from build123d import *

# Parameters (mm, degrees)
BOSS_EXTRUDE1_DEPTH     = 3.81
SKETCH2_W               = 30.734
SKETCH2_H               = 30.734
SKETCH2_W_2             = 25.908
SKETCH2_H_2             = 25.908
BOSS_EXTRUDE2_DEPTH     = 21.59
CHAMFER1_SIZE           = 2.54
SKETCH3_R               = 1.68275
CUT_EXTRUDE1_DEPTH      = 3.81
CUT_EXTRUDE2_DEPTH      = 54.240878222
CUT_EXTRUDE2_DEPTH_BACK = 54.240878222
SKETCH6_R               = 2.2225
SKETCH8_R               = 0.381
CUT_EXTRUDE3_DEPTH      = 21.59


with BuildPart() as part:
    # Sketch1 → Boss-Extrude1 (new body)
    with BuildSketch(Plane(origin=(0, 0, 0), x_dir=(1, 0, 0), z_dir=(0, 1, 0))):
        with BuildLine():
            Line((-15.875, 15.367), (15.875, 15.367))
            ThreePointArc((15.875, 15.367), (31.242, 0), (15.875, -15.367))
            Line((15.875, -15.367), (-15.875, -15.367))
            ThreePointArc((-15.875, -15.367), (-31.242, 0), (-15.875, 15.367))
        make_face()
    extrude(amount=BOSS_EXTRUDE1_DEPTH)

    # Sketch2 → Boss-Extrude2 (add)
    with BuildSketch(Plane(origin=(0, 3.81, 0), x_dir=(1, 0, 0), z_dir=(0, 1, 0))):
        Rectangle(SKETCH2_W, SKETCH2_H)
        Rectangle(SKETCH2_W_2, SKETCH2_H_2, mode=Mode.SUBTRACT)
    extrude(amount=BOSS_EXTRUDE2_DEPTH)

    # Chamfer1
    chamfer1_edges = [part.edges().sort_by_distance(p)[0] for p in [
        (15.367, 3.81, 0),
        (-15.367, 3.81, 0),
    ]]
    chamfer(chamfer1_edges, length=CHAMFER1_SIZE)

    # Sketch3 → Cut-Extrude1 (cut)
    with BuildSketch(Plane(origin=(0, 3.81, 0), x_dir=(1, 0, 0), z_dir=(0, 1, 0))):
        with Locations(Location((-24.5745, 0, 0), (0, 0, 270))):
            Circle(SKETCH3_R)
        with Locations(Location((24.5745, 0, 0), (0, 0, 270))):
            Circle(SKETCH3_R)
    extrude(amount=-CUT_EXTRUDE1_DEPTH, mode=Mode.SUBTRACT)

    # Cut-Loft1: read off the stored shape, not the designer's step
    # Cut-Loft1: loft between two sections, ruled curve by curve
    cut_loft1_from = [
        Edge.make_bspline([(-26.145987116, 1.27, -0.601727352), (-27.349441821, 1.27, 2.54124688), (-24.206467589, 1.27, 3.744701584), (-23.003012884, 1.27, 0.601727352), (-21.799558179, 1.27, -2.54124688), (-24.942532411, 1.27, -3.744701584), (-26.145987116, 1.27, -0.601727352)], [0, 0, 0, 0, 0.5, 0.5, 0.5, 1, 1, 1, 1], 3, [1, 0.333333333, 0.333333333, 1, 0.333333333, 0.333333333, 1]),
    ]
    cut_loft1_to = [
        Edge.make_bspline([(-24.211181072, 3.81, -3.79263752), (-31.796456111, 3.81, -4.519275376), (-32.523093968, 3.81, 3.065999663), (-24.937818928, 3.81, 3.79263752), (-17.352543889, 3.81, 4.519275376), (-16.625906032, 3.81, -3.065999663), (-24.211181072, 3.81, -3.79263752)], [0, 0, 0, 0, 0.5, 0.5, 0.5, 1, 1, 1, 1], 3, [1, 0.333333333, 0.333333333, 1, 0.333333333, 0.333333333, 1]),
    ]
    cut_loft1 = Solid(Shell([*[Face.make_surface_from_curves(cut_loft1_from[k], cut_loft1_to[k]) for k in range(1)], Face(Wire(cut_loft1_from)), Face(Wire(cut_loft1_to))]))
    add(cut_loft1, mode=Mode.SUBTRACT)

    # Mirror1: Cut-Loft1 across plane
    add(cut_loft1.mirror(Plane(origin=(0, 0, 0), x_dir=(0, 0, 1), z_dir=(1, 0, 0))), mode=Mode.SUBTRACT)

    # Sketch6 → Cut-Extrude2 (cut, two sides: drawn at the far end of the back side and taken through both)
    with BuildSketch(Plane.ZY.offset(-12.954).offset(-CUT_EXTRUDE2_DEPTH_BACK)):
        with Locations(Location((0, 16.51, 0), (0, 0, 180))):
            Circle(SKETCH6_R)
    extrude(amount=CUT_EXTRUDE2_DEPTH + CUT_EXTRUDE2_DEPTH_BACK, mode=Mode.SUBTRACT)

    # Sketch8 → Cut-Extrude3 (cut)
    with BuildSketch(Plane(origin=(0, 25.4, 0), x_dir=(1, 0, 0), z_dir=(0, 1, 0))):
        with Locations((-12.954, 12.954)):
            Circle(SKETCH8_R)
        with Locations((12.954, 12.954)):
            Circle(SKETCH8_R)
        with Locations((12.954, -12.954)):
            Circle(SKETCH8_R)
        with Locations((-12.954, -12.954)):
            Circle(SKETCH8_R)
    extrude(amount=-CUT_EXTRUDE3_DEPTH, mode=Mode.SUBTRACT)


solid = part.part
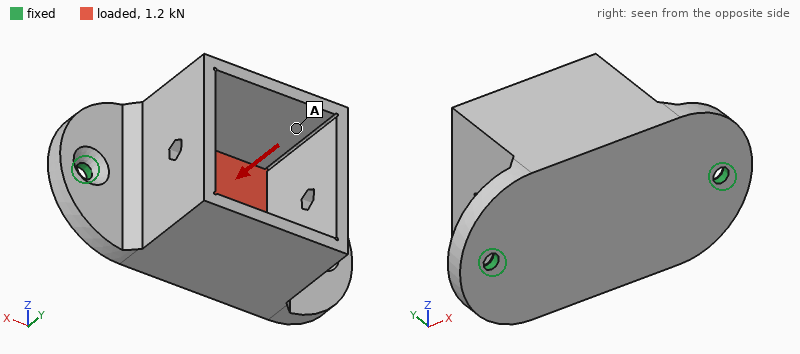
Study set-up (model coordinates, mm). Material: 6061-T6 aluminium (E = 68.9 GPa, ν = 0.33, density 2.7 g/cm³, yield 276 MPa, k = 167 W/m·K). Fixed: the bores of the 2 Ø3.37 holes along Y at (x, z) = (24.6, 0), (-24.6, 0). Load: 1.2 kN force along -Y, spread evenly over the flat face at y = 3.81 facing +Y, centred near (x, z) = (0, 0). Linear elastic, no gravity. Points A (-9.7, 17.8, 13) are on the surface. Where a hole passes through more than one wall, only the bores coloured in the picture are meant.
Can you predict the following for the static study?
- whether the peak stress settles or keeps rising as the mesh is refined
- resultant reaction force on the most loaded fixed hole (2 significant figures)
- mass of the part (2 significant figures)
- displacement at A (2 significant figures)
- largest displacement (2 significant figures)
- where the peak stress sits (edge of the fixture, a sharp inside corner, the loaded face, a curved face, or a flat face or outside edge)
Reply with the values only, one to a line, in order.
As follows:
keeps rising
830 N
34 g
27 µm
41 µm
edge of the fixture
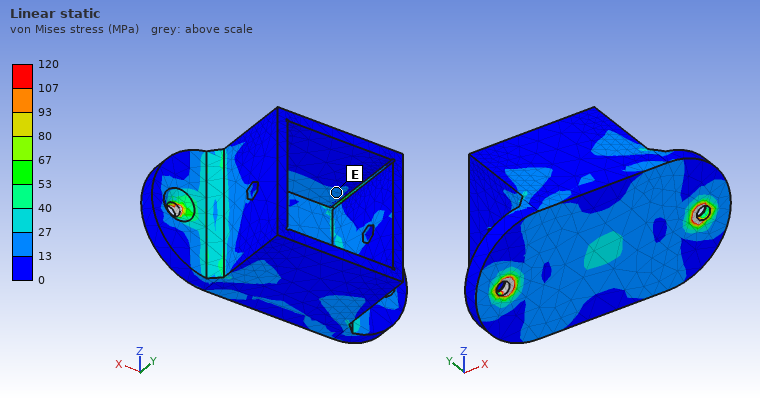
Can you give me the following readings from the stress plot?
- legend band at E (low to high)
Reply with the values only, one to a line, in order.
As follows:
13 to 27 MPa
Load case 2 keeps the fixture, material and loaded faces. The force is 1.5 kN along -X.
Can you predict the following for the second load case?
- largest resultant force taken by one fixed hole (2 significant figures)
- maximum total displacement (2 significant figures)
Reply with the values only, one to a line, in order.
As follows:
760 N
4.0 µm
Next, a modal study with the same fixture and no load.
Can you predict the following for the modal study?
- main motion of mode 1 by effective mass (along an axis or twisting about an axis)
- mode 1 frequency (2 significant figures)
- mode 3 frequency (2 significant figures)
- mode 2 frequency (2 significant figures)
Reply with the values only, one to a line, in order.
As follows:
along Z
2200 Hz
6400 Hz
6300 Hz
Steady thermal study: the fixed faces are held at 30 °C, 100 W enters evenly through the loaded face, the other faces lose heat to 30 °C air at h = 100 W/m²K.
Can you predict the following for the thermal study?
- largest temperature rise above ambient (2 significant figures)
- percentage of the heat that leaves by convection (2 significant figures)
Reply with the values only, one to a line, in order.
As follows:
53 K
27 %
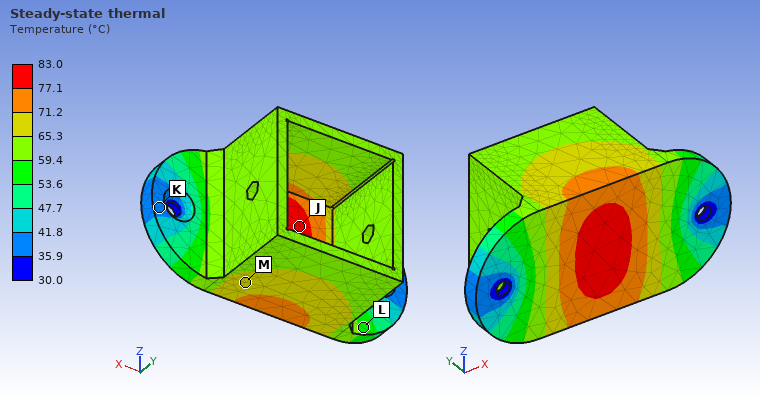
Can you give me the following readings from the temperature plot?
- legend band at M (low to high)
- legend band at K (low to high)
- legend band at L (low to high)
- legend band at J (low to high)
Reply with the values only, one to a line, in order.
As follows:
65.3 to 71.2 °C
35.9 to 41.8 °C
53.6 to 59.4 °C
77.1 to 83.0 °C
